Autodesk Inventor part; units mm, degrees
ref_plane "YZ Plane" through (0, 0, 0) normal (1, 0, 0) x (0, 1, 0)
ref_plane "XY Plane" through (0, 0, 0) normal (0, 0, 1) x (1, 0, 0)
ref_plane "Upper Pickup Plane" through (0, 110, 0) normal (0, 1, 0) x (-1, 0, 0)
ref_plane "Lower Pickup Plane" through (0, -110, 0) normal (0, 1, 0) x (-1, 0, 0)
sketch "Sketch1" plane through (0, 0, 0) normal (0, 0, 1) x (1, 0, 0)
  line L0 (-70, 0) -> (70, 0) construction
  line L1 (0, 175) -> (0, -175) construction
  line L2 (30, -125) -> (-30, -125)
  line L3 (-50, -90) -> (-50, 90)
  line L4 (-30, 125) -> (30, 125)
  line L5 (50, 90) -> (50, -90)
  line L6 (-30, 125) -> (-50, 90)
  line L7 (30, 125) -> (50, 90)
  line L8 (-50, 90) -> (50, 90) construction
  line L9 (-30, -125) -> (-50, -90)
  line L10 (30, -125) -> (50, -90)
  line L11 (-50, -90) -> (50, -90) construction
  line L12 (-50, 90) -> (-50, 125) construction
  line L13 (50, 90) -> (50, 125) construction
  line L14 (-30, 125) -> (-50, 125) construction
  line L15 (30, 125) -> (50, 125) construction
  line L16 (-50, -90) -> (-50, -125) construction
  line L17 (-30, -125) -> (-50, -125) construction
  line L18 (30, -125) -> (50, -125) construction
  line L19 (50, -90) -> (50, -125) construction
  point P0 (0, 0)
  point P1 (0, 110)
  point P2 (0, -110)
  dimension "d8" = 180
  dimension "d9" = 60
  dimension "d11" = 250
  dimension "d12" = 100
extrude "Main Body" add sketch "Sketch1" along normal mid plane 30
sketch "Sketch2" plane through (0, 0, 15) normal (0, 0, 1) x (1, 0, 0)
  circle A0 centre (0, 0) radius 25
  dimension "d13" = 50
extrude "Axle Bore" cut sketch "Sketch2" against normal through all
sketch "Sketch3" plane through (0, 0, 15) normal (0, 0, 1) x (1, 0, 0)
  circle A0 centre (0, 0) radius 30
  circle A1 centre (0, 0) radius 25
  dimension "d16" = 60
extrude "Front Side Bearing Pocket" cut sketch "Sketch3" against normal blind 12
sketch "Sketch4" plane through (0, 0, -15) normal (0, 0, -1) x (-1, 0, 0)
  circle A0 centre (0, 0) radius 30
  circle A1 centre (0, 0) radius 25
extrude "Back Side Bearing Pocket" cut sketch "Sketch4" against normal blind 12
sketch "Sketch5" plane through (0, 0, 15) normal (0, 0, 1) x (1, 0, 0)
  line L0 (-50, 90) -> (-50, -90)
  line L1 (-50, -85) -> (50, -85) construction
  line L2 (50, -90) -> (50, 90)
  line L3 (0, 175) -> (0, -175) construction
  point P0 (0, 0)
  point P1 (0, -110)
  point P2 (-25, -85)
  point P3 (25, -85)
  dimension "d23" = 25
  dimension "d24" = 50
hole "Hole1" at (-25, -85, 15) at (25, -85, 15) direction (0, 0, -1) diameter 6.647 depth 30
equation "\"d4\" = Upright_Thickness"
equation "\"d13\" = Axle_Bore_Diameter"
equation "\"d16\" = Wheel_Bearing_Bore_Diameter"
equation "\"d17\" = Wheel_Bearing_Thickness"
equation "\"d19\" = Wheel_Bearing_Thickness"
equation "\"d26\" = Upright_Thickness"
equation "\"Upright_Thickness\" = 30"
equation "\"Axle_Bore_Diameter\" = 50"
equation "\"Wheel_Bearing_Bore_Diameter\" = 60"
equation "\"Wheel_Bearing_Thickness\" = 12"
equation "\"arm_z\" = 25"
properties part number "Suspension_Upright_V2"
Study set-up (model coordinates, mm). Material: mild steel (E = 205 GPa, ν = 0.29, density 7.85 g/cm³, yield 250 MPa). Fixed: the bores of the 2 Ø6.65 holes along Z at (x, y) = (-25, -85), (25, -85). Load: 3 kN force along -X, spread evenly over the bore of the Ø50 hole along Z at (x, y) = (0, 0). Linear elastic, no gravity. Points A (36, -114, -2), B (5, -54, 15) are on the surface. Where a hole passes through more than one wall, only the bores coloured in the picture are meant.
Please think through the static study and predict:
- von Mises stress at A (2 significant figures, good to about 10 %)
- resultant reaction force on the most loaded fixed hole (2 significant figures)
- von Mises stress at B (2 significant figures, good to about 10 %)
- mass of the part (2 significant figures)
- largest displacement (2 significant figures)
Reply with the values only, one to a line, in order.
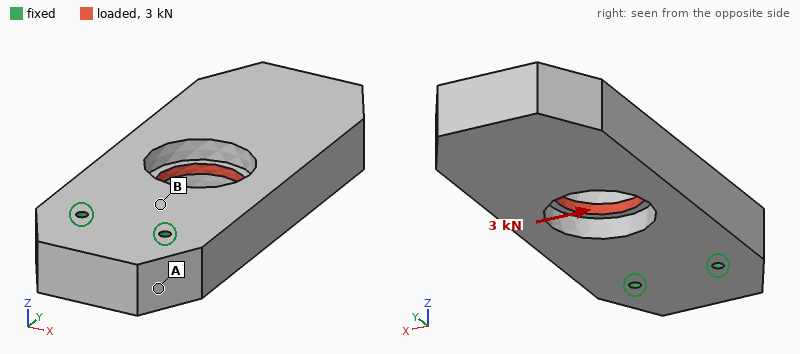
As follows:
1.2 MPa
5.0 kN
4.4 MPa
4.9 kg
11 µm
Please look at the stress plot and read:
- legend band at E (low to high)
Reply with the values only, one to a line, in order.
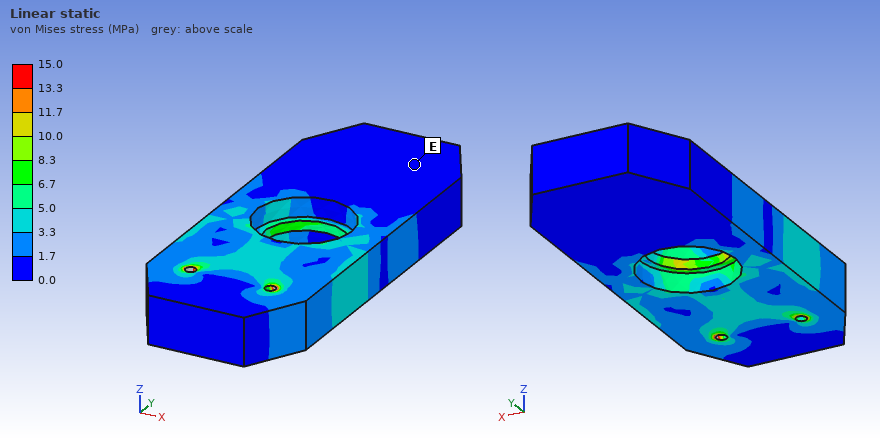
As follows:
0.0 to 1.7 MPa
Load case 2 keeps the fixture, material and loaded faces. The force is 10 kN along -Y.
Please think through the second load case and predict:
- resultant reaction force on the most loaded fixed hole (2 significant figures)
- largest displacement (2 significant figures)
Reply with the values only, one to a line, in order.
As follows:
5.0 kN
3.4 µm
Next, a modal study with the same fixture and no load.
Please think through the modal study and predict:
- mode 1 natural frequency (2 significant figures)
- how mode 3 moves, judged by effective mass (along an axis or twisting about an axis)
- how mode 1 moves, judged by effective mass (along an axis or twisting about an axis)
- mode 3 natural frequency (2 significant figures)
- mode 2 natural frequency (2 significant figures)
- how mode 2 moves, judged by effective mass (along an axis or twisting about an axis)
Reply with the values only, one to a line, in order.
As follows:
480 Hz
twisting about Y
along Z
1900 Hz
1300 Hz
along X
